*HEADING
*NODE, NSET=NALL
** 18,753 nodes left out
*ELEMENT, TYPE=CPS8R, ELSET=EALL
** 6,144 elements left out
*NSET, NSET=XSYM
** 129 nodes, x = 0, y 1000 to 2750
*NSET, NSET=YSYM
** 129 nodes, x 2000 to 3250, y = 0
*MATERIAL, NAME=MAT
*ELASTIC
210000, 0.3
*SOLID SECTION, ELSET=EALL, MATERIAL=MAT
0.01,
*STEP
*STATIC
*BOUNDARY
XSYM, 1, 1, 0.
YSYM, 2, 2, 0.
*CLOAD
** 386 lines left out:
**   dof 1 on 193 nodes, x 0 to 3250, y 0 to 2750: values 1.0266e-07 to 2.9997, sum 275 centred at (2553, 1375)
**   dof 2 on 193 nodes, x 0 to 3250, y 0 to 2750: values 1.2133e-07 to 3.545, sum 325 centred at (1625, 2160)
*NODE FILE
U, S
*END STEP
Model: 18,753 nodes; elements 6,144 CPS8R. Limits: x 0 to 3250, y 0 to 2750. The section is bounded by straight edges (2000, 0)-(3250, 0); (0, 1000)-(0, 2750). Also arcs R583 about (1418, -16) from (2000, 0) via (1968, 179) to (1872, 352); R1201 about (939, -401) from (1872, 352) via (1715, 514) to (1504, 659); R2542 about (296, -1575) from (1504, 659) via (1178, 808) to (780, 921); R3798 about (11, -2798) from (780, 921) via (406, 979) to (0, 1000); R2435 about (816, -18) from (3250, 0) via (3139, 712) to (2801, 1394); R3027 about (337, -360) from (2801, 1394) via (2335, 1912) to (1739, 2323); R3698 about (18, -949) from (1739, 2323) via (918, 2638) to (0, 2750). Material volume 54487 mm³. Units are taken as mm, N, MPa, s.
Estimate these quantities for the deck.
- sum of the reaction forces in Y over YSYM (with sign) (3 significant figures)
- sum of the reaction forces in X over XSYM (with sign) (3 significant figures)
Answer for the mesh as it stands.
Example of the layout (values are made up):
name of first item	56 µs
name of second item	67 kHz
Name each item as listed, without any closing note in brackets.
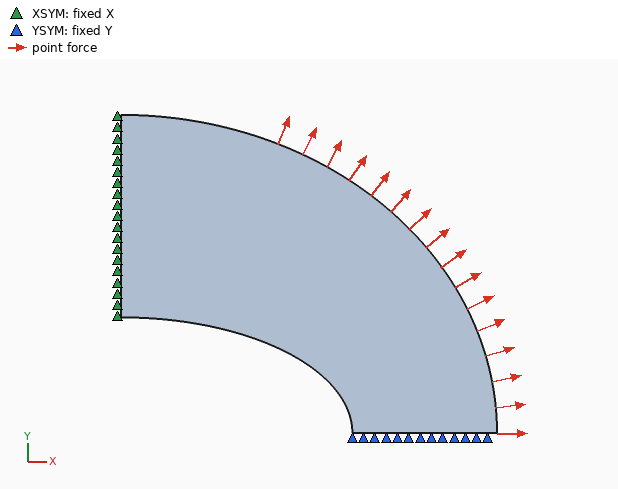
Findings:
sum of the reaction forces in Y over YSYM (with sign)	-325 N
sum of the reaction forces in X over XSYM (with sign)	-275 N
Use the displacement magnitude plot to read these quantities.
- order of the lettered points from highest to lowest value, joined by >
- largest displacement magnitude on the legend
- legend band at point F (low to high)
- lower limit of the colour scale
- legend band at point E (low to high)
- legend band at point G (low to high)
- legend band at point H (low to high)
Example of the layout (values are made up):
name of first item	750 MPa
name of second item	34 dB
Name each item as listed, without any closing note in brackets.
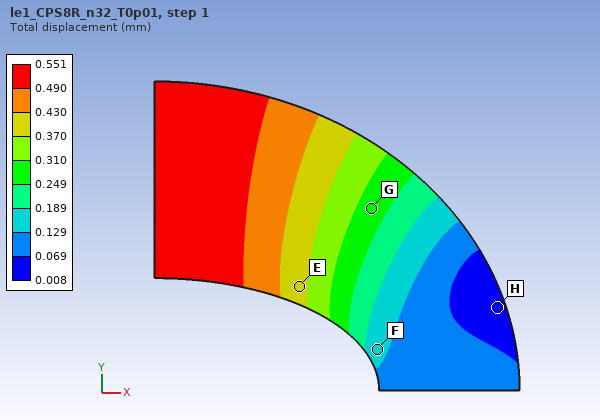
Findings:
order of the lettered points from highest to lowest value, joined by >	E > G > F > H
largest displacement magnitude on the legend	0.551 mm
legend band at point F	0.129 to 0.189 mm
lower limit of the colour scale	0.008 mm
legend band at point E	0.370 to 0.430 mm
legend band at point G	0.249 to 0.310 mm
legend band at point H	0.008 to 0.069 mm
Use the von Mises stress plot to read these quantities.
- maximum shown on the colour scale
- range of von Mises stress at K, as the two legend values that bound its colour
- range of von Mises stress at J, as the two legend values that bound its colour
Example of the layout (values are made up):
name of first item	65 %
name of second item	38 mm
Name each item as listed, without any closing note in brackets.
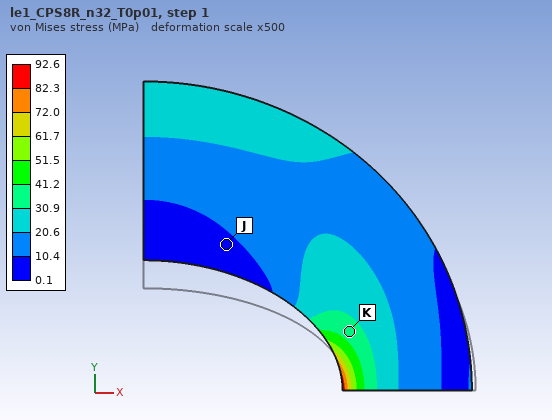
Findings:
maximum shown on the colour scale	92.6 MPa
range of von Mises stress at K, as the two legend values that bound its colour	30.9 to 41.2 MPa
range of von Mises stress at J, as the two legend values that bound its colour	0.1 to 10.4 MPa
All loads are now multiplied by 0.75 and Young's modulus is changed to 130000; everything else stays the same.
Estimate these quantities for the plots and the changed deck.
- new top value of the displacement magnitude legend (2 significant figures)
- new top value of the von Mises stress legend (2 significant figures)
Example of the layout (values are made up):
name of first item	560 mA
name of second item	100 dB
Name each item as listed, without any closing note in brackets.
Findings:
new top value of the displacement magnitude legend	0.67 mm
new top value of the von Mises stress legend	69 MPa
